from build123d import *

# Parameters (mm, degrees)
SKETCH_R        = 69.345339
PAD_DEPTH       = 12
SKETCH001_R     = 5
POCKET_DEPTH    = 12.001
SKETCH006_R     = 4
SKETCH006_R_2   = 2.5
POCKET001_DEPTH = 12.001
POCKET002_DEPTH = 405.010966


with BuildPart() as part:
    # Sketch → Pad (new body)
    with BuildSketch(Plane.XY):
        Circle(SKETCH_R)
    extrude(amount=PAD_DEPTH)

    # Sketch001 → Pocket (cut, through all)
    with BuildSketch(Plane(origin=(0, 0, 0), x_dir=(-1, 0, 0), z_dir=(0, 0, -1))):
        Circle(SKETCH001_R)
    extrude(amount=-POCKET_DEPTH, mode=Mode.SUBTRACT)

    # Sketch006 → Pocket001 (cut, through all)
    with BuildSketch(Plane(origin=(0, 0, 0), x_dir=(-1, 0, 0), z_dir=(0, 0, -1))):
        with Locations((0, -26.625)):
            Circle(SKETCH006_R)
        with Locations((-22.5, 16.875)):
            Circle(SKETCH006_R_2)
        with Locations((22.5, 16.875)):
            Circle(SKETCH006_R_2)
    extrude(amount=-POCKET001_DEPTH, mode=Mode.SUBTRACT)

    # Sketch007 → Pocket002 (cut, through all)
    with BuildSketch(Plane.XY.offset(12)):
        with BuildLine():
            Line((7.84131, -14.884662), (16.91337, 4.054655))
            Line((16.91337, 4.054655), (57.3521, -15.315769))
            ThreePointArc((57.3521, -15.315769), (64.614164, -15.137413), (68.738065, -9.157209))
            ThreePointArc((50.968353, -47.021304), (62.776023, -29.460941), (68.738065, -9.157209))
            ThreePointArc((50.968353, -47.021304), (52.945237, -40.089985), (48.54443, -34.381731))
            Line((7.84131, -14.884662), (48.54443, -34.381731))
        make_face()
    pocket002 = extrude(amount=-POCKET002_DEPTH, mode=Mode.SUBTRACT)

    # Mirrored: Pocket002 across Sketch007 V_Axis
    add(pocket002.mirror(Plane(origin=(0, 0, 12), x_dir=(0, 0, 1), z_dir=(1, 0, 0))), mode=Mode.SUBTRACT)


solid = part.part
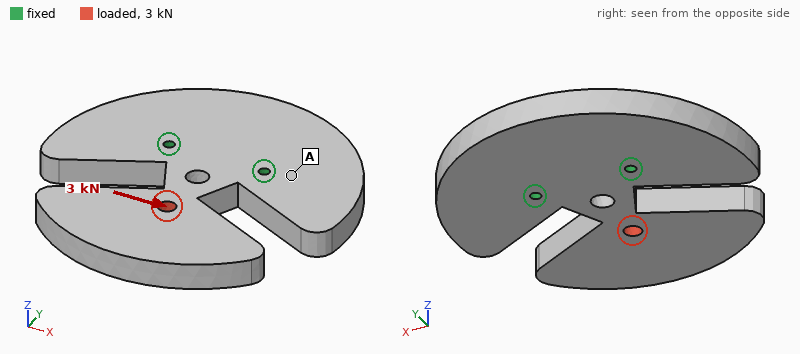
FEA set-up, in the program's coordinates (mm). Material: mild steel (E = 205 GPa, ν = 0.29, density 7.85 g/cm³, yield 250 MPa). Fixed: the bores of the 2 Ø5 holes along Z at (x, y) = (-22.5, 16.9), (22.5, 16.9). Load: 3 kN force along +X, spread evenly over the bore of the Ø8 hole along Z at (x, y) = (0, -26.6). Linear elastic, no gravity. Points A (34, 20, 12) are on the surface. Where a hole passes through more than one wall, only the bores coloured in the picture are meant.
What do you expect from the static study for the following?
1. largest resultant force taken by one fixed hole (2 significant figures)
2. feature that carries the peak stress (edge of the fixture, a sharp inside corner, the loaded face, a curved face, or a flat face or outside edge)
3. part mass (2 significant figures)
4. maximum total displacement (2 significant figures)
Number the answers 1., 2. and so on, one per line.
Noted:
1. 3.3 kN
2. a flat face or outside edge
3. 1.2 kg
4. 58 µm
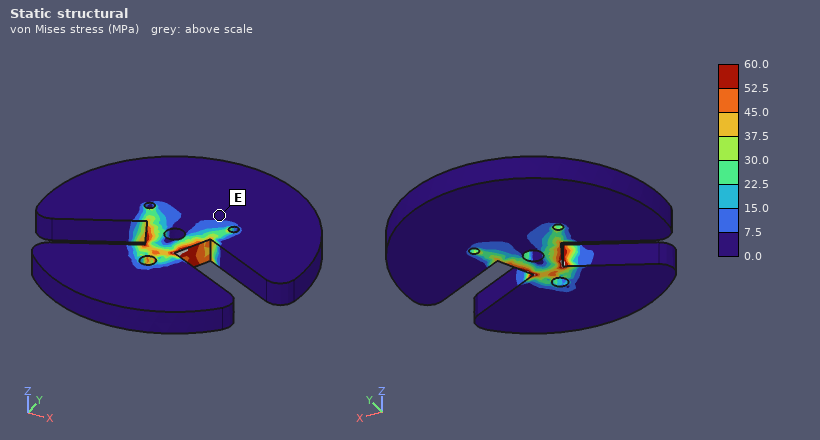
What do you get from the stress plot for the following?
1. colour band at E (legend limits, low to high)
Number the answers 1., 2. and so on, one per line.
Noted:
1. 0.0 to 7.5 MPa
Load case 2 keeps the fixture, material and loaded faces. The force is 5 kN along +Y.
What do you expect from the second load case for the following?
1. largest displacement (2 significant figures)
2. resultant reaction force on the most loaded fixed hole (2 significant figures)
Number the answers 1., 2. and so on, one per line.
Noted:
1. 5.9 µm
2. 2.6 kN
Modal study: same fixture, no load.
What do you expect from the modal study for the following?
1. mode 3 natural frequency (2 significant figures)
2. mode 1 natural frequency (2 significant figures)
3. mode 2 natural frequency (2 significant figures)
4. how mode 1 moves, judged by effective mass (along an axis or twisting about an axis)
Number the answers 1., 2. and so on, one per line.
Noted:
1. 1300 Hz
2. 720 Hz
3. 1300 Hz
4. along Z
